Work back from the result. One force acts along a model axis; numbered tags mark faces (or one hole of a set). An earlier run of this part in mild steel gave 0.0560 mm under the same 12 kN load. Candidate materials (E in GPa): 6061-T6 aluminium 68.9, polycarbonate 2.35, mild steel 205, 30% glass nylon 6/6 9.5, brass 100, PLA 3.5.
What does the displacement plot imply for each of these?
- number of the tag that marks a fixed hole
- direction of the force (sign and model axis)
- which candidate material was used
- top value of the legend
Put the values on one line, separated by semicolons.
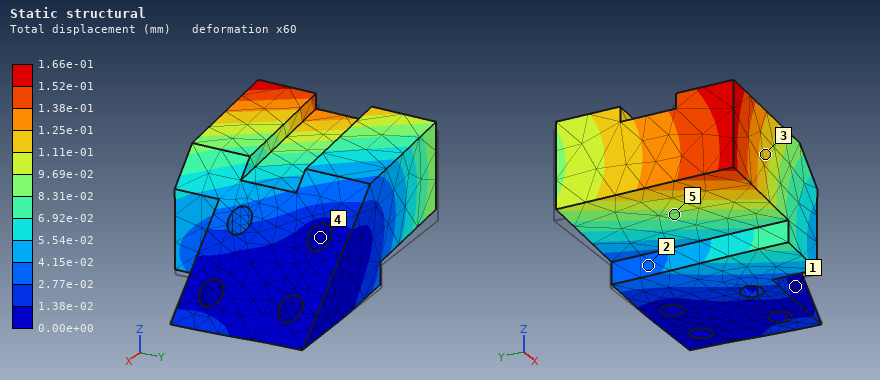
4; +Z; 6061-T6 aluminium; 1.66e-01 mm
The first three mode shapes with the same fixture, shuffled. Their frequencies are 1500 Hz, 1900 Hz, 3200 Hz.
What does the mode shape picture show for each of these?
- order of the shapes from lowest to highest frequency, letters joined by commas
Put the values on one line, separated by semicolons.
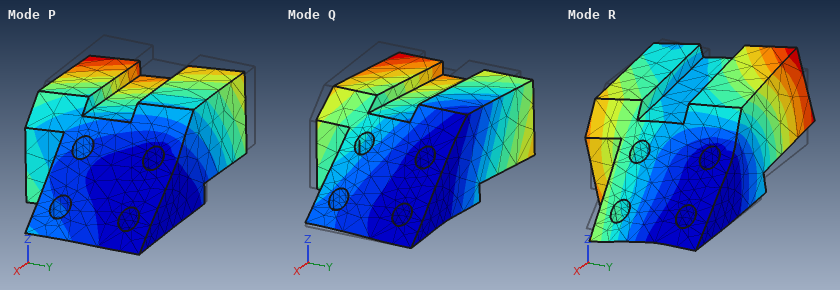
Q, P, R
